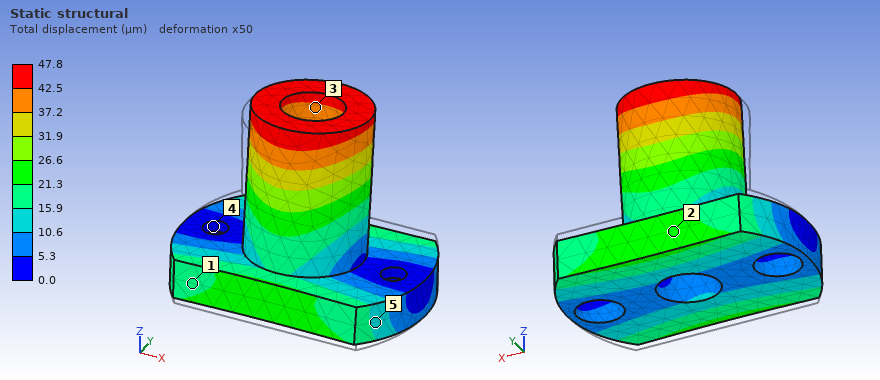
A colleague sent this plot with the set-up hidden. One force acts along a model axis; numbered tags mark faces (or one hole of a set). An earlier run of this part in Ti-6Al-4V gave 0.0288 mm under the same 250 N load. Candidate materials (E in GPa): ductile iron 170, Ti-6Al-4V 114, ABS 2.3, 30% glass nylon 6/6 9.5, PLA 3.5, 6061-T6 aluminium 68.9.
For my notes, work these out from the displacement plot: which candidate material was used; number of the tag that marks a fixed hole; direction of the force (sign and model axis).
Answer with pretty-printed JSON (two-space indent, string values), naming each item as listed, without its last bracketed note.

{
  "which candidate material was used": "6061-T6 aluminium",
  "number of the tag that marks a fixed hole": "4",
  "direction of the force": "+Y"
}
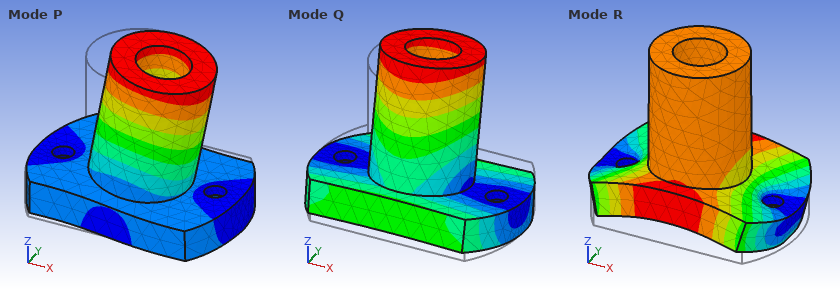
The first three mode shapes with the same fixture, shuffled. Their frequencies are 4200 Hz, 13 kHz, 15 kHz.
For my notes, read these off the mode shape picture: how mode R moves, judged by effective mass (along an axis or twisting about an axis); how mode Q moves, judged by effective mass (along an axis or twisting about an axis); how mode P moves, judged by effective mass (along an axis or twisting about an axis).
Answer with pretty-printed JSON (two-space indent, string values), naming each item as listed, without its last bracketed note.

{
  "how mode R moves, judged by effective mass": "along Z",
  "how mode Q moves, judged by effective mass": "along Y",
  "how mode P moves, judged by effective mass": "along X"
}
